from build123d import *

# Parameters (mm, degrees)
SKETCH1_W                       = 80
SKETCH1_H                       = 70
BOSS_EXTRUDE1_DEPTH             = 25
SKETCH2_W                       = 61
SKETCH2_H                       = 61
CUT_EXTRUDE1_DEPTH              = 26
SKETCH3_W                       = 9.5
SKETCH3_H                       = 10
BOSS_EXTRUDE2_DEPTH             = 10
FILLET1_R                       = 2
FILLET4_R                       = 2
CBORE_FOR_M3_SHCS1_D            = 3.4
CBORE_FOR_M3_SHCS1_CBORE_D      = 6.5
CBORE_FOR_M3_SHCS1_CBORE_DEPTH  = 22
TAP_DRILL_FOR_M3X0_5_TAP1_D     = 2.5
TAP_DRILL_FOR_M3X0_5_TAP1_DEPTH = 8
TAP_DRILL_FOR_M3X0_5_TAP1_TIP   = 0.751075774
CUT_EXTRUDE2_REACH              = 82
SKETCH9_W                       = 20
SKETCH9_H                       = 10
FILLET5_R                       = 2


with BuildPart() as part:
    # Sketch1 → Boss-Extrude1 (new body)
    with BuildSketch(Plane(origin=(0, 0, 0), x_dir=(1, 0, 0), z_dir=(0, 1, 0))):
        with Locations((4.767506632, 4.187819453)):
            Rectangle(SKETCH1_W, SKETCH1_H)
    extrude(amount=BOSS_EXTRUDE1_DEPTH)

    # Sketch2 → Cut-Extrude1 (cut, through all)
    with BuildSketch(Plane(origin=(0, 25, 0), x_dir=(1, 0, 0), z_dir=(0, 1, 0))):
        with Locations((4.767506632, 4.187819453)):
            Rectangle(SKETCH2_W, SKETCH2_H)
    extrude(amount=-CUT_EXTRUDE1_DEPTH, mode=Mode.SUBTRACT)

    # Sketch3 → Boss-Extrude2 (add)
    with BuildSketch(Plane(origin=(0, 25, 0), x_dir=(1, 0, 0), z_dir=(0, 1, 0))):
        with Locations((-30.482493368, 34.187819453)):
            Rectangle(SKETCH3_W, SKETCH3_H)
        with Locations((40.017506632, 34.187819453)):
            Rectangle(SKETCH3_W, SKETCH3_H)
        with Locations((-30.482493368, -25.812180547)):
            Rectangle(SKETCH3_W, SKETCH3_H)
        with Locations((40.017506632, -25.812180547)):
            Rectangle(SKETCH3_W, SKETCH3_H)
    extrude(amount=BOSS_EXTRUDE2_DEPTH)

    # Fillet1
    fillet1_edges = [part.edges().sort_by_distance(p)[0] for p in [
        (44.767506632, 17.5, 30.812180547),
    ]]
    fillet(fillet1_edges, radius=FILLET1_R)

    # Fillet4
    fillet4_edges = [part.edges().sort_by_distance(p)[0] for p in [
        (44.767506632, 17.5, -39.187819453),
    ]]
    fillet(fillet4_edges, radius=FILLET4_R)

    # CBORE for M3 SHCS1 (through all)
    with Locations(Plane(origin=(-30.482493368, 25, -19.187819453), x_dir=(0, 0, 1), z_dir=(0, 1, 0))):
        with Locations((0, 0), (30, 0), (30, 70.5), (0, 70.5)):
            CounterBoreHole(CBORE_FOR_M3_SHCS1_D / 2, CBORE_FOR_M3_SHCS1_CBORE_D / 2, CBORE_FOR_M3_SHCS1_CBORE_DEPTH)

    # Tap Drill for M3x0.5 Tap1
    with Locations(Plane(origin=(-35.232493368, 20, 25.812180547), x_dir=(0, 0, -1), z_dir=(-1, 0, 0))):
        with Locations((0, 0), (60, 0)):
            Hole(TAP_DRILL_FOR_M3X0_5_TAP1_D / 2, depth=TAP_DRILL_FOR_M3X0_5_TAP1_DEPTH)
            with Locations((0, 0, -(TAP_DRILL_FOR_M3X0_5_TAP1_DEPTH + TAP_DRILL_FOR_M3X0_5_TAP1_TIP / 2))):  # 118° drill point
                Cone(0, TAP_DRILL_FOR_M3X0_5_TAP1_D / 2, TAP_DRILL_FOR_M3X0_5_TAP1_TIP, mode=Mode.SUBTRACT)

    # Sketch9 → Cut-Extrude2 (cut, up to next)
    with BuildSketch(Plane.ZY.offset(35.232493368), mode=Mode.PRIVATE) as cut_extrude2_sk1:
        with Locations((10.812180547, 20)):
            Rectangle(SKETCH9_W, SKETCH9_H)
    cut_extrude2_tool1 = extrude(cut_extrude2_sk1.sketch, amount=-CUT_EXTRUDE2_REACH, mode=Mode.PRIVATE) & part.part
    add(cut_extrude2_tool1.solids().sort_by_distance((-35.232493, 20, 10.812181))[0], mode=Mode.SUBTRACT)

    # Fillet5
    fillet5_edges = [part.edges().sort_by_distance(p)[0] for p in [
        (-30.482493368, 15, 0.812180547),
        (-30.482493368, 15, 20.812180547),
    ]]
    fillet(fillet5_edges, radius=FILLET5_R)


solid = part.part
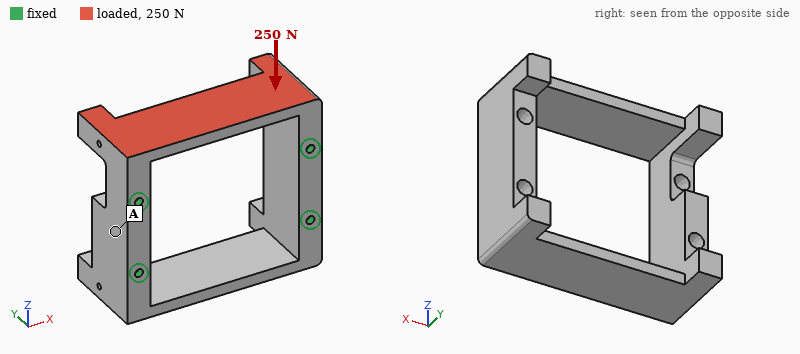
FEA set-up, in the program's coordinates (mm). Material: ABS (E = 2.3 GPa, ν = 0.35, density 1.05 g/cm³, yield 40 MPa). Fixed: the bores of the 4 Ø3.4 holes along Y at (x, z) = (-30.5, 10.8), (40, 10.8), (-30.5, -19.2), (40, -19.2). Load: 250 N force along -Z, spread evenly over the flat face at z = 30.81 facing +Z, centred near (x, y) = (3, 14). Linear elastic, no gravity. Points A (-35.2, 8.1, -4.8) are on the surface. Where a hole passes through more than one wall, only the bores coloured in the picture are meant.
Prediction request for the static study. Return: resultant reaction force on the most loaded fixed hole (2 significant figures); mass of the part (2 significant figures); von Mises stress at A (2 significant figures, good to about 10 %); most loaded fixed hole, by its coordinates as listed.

100 N
48 g
1.3 MPa
(40, 10.8)
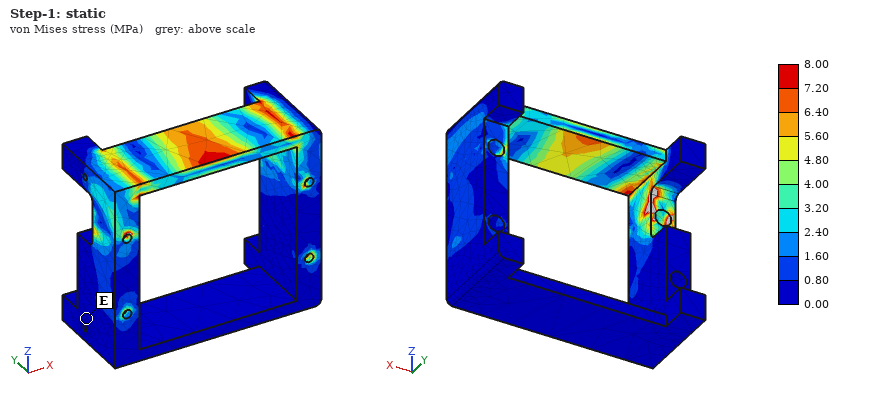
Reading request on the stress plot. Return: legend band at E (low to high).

0.00 to 0.80 MPa
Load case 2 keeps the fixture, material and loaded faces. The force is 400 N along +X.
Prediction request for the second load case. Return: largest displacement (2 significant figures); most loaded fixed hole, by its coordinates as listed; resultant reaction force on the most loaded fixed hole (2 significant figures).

0.49 mm
(40, 10.8)
290 N
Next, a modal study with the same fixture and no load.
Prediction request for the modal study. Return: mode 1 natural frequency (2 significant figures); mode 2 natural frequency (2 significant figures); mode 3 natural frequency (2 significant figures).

1300 Hz
1400 Hz
1400 Hz
